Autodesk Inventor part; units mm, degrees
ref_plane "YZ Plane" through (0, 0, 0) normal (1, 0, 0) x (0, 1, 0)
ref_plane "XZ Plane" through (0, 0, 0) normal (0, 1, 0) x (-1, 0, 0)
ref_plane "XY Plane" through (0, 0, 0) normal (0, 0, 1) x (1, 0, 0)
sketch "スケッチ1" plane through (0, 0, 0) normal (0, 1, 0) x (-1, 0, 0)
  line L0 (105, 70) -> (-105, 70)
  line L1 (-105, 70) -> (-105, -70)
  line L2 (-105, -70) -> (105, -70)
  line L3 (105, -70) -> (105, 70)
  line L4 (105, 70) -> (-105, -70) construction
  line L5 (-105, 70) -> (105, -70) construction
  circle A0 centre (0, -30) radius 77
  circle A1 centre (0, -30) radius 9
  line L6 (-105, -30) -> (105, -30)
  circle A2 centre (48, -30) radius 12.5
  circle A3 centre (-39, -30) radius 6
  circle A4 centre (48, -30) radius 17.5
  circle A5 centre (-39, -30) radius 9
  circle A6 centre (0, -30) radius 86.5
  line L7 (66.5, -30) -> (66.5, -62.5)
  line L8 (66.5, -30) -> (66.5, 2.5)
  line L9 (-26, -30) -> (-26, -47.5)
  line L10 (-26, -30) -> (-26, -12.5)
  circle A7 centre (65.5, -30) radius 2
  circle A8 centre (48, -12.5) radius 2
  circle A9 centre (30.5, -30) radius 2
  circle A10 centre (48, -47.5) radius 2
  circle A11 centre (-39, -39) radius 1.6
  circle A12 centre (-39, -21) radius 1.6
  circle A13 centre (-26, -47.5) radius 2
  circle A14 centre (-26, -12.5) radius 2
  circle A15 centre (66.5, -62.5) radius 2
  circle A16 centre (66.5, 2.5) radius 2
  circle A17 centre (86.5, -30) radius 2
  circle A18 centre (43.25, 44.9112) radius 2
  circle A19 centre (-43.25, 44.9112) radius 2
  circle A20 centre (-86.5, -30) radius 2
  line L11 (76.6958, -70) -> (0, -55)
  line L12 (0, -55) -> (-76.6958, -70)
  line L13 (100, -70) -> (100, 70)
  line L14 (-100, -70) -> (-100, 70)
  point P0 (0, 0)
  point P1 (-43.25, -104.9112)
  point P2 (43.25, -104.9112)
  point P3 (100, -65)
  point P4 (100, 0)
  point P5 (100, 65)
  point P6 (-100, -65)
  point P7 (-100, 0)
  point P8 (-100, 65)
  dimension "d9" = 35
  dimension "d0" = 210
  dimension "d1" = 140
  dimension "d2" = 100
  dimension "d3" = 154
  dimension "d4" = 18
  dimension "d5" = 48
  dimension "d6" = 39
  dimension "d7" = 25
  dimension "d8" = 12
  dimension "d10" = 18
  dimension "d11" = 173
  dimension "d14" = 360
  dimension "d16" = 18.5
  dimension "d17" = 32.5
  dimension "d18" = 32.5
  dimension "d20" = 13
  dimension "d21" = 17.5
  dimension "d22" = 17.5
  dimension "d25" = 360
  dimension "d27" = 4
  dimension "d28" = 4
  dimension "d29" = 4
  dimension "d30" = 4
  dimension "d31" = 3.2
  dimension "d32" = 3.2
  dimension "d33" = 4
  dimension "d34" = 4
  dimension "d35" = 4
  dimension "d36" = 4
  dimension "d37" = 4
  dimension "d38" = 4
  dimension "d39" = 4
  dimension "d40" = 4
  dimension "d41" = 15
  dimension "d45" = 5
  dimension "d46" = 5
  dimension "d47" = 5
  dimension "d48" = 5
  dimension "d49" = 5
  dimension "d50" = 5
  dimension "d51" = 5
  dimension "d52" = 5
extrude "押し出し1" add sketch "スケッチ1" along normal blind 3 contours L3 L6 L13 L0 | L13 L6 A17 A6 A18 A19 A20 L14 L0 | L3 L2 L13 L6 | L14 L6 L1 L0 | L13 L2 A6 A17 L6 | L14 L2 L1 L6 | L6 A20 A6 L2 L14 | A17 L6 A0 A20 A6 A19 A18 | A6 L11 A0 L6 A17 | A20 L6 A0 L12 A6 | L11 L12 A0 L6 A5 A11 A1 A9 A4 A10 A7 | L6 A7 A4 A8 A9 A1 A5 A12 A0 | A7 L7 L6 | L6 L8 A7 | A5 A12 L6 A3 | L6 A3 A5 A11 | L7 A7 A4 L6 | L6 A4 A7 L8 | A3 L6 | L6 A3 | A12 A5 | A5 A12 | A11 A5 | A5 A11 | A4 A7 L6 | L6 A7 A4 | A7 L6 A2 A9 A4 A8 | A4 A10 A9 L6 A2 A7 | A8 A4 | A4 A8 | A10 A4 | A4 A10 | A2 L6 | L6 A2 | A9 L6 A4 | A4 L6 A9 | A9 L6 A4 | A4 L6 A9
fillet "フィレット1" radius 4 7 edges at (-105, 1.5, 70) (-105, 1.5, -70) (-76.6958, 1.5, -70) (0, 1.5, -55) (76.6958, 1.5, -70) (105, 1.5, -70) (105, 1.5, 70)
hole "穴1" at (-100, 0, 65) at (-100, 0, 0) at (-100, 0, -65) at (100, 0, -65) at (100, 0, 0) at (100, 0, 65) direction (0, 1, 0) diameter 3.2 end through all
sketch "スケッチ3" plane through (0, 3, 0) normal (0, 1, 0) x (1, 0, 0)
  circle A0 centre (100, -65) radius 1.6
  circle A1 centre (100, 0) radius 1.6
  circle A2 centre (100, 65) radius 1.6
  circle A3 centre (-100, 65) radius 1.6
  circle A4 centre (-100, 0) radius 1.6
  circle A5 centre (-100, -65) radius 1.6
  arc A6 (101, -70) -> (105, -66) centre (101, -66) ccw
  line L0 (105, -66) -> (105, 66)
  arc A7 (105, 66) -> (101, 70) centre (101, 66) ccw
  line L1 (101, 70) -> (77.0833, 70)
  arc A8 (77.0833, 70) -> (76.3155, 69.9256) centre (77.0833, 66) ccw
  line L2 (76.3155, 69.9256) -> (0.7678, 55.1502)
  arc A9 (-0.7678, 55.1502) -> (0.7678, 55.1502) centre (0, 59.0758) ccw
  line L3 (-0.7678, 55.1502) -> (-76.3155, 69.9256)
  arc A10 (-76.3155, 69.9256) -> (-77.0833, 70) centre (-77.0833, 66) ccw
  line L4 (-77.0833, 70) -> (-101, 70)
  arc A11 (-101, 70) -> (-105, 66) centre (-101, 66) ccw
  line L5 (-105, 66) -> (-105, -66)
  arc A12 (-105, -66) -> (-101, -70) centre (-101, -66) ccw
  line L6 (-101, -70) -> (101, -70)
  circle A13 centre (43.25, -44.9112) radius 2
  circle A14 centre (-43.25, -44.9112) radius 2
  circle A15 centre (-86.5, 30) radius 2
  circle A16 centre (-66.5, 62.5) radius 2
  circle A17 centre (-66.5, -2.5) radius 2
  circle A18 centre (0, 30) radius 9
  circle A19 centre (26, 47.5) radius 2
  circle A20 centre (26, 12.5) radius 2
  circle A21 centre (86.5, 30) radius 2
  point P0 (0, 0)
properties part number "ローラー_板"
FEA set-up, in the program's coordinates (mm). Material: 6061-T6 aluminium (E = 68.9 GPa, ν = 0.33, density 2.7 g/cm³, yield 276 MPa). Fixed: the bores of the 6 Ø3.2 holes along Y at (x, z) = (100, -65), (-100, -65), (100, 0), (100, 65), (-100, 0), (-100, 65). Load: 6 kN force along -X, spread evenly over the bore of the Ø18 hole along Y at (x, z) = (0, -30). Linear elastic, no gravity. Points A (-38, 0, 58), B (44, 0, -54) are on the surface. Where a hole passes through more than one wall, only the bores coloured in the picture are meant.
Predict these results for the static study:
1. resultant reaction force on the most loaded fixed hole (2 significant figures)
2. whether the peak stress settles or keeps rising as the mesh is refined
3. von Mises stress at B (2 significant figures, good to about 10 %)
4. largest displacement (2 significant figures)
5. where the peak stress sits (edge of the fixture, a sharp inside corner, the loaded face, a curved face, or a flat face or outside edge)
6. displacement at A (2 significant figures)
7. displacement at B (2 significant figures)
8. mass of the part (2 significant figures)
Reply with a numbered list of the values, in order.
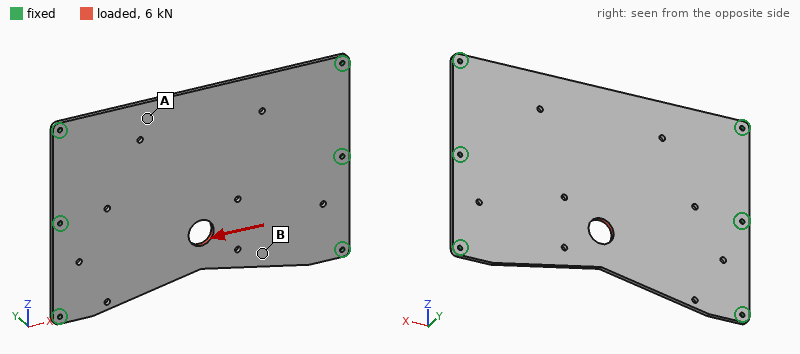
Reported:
1. 1.4 kN
2. keeps rising
3. 13 MPa
4. 29 µm
5. edge of the fixture
6. 5.9 µm
7. 15 µm
8. 230 g
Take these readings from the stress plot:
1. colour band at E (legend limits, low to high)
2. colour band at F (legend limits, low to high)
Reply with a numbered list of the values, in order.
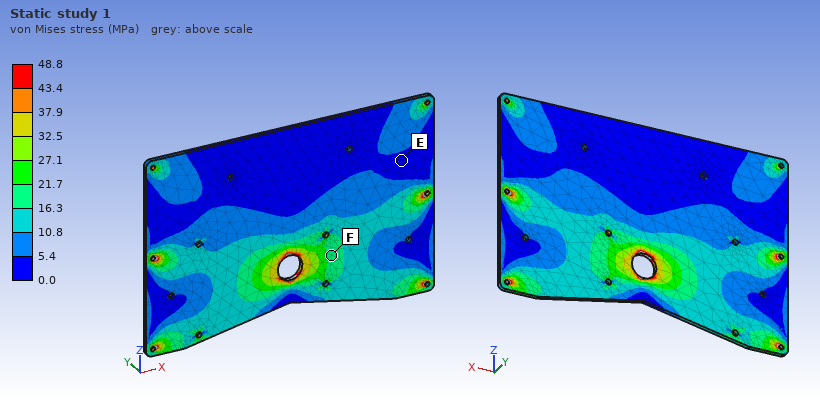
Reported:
1. 0.0 to 5.4 MPa
2. 16.3 to 21.7 MPa
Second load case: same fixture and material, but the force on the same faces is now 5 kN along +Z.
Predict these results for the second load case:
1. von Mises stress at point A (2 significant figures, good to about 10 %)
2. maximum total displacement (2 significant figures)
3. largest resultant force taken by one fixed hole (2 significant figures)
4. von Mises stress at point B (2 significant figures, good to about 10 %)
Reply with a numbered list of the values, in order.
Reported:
1. 7.5 MPa
2. 50 µm
3. 1.2 kN
4. 6.0 MPa
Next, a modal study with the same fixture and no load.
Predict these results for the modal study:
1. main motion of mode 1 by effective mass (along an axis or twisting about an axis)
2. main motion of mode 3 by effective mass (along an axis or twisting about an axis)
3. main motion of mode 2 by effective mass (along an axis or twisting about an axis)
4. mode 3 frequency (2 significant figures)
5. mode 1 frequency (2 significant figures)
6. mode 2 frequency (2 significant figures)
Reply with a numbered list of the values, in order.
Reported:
1. along Y
2. twisting about Z
3. twisting about X
4. 960 Hz
5. 340 Hz
6. 540 Hz
